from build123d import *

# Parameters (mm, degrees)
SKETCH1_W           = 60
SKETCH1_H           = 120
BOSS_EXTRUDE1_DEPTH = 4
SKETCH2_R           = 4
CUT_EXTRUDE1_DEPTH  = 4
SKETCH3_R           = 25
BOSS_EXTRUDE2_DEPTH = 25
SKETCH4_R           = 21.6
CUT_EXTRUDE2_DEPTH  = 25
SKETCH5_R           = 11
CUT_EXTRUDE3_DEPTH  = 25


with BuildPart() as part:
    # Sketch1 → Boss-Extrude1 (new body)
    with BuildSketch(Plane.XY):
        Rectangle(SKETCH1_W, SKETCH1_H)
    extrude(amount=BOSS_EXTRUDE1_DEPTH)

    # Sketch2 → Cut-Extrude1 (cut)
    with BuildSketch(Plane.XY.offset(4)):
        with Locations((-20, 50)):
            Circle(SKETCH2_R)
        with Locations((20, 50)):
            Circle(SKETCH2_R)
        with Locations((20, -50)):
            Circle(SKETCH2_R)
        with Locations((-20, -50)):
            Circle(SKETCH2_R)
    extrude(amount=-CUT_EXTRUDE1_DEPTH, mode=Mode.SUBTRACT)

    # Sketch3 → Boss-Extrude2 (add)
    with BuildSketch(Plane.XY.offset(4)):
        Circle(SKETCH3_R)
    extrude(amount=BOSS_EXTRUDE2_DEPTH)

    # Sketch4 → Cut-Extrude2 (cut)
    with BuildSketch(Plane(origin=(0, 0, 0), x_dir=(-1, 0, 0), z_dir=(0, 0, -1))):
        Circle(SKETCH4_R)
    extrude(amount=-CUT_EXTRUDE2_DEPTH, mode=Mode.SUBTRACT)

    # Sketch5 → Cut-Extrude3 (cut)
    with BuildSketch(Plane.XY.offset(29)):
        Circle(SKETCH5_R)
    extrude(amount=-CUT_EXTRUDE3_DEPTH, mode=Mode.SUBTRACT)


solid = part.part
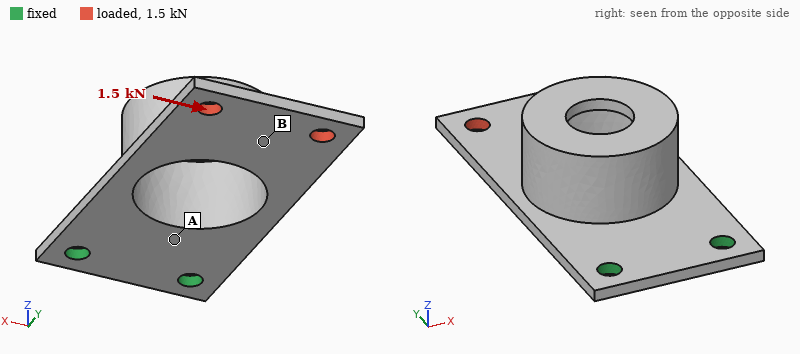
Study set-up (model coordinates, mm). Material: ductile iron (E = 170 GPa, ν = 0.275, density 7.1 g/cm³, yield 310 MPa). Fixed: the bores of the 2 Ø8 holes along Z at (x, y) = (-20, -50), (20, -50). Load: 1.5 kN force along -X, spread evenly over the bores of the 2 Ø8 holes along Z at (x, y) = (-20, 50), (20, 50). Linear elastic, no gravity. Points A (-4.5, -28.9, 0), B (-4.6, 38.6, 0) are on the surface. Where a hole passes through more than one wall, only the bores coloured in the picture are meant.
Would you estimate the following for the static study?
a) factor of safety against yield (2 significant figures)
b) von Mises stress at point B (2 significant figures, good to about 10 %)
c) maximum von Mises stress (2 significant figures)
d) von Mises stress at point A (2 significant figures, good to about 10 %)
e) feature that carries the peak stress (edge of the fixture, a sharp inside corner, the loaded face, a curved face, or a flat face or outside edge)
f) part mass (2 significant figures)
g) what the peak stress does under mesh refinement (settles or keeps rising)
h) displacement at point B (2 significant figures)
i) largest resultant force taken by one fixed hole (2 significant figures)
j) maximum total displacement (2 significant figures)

2.4
20 MPa
130 MPa
45 MPa
a flat face or outside edge
280 g
settles
0.095 mm
3.5 kN
0.12 mm
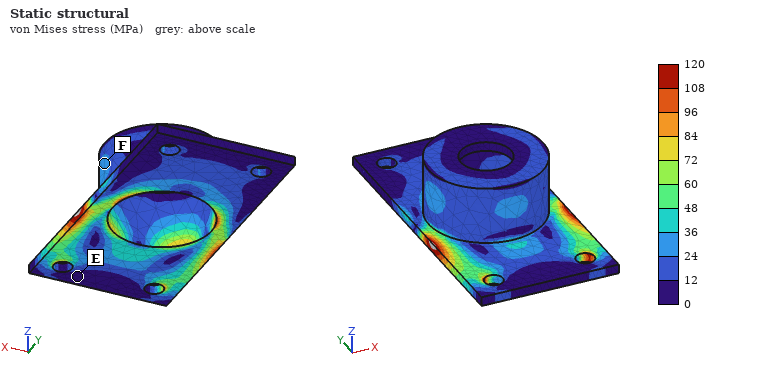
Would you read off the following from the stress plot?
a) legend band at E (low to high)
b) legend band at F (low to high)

0 to 12 MPa
24 to 36 MPa
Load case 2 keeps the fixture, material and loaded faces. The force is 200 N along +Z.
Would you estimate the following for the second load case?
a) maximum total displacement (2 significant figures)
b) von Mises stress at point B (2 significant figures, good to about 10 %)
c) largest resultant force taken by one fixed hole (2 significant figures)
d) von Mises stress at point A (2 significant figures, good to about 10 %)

0.93 mm
14 MPa
140 N
92 MPa
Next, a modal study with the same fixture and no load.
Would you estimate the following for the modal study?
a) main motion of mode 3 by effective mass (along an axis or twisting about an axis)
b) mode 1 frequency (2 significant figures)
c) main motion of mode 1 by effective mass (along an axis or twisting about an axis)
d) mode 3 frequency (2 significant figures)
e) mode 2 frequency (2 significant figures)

along X
270 Hz
along Z
2000 Hz
1200 Hz
